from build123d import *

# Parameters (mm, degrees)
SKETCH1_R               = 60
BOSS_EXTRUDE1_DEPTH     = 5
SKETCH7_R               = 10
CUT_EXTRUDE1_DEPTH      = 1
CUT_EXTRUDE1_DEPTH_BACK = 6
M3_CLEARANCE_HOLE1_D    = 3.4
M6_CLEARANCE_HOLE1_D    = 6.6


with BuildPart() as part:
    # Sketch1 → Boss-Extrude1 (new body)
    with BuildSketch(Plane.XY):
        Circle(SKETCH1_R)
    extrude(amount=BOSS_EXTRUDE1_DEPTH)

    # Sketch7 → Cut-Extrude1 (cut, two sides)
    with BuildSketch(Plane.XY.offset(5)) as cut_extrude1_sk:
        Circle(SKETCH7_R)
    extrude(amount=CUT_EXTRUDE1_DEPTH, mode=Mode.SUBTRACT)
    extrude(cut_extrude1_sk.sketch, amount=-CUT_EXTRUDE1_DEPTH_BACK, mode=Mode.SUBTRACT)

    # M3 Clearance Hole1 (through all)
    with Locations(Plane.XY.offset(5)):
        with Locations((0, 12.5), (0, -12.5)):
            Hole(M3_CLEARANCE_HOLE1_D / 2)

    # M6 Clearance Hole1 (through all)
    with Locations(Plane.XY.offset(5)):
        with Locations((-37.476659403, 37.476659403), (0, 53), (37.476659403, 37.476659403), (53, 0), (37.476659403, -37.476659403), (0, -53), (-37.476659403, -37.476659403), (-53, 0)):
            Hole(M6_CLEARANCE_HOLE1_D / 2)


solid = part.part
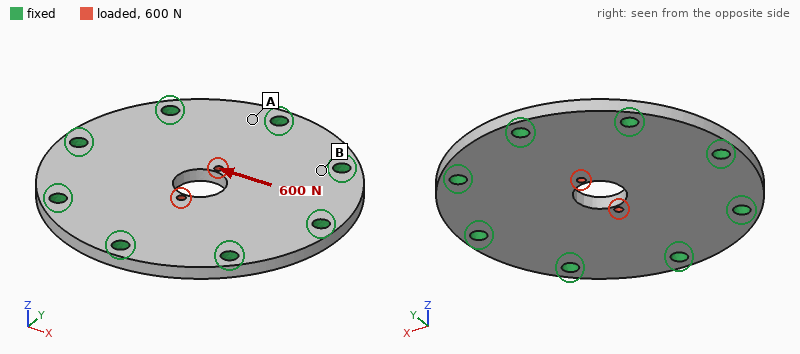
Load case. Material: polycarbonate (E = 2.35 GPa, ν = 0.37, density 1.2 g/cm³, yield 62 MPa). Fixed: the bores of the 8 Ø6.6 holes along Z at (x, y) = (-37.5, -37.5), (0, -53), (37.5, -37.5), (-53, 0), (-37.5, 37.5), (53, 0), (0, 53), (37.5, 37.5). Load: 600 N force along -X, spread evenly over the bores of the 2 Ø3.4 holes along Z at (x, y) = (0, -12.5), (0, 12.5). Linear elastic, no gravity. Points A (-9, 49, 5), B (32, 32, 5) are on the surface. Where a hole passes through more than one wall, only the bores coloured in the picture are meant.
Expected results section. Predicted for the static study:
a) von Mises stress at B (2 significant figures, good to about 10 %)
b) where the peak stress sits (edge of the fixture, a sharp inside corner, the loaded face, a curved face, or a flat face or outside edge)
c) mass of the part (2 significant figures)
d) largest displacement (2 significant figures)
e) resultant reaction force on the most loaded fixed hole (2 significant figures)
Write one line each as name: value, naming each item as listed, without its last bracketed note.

von Mises stress at B: 1.3 MPa
where the peak stress sits: the loaded face
mass of the part: 64 g
largest displacement: 36 µm
resultant reaction force on the most loaded fixed hole: 110 N
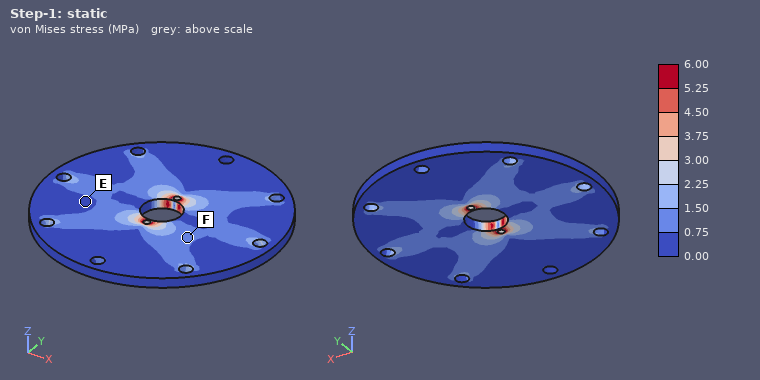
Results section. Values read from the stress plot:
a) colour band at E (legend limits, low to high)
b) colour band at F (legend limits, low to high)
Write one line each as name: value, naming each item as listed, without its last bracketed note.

colour band at E: 0.00 to 0.75 MPa
colour band at F: 0.75 to 1.50 MPa
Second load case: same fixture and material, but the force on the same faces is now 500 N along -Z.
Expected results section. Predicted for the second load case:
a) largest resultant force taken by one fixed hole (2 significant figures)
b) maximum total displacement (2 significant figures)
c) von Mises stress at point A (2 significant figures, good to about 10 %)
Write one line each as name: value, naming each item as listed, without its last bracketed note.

largest resultant force taken by one fixed hole: 79 N
maximum total displacement: 1.3 mm
von Mises stress at point A: 6.9 MPa
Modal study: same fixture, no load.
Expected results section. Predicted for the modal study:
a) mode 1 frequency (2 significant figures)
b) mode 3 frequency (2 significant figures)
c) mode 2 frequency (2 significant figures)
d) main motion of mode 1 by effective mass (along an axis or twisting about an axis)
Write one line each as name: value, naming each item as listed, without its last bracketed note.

mode 1 frequency: 1100 Hz
mode 3 frequency: 2200 Hz
mode 2 frequency: 2200 Hz
main motion of mode 1 by effective mass: along Z
